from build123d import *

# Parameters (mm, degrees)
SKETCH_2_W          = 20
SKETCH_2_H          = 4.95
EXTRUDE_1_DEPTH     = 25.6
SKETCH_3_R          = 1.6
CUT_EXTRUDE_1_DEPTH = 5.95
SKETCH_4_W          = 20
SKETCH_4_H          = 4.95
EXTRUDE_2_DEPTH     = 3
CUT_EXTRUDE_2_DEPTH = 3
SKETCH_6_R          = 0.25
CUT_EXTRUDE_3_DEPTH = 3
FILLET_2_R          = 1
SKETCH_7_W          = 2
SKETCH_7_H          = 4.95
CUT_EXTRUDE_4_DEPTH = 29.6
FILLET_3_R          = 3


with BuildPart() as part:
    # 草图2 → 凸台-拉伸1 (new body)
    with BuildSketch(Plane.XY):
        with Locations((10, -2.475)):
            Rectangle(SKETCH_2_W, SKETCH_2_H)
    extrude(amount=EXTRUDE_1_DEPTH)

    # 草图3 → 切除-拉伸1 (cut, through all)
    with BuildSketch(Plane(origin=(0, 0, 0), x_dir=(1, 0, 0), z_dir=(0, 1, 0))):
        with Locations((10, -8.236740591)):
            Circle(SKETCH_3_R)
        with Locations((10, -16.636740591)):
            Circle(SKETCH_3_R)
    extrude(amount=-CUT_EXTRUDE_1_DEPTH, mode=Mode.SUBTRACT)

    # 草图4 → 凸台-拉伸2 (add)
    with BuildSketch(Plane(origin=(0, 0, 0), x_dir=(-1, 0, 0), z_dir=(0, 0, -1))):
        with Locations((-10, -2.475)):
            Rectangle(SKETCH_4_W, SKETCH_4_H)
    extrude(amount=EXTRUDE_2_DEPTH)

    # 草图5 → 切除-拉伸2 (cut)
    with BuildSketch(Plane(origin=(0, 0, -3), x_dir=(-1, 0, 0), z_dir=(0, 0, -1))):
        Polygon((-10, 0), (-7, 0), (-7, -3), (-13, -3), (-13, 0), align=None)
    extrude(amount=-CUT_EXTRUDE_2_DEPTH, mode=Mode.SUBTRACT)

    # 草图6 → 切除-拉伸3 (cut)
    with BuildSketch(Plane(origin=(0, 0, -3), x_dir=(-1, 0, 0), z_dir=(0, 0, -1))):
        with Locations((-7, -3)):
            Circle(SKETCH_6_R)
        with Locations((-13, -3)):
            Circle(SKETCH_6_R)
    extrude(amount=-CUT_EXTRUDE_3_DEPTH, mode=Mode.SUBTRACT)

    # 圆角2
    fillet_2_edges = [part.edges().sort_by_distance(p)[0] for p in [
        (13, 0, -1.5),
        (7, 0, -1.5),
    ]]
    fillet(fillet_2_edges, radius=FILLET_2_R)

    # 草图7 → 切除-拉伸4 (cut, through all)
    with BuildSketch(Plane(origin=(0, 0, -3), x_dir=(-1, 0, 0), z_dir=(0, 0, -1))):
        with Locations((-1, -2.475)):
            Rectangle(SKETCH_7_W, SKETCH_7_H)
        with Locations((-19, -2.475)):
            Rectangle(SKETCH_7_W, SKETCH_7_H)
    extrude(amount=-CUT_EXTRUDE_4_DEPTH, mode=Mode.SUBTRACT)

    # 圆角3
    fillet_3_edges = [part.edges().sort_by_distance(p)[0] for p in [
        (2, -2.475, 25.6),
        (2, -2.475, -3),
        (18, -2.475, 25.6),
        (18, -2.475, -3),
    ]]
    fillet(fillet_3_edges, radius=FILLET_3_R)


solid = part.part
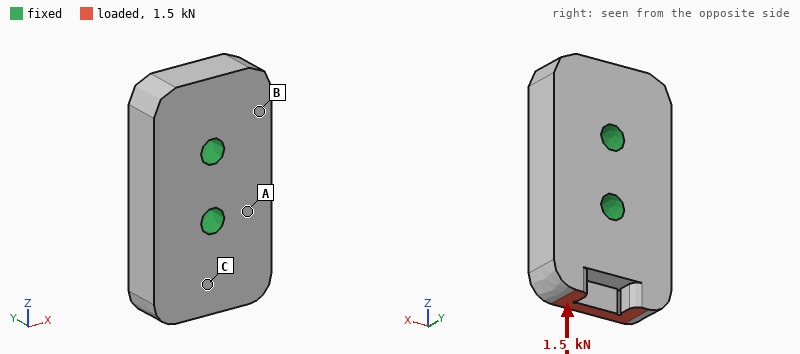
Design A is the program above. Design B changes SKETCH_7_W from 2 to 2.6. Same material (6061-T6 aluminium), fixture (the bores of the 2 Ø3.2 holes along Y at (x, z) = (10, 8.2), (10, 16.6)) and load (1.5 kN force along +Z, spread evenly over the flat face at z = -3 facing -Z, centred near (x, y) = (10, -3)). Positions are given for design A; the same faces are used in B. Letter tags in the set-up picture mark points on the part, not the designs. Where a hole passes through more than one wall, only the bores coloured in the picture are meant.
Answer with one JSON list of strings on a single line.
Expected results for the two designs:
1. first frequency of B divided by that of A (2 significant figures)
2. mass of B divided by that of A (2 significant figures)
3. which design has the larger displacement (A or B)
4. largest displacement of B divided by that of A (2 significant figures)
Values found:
["1.0", "0.96", "B", "1.1"]
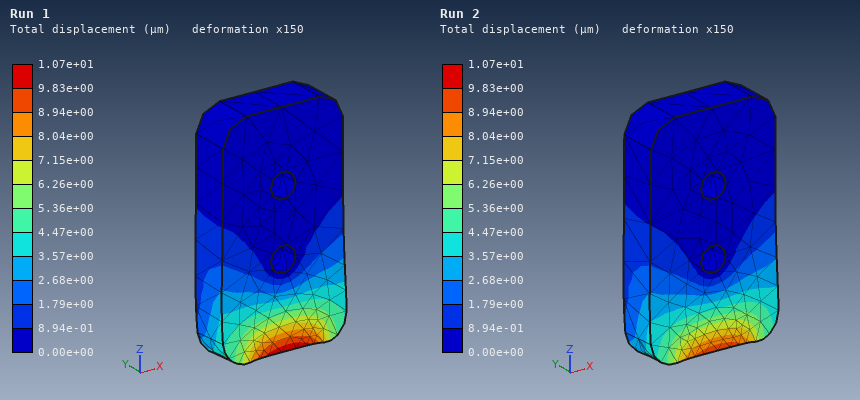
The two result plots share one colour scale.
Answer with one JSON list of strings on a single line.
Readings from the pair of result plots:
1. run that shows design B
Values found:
["Run 1"]
